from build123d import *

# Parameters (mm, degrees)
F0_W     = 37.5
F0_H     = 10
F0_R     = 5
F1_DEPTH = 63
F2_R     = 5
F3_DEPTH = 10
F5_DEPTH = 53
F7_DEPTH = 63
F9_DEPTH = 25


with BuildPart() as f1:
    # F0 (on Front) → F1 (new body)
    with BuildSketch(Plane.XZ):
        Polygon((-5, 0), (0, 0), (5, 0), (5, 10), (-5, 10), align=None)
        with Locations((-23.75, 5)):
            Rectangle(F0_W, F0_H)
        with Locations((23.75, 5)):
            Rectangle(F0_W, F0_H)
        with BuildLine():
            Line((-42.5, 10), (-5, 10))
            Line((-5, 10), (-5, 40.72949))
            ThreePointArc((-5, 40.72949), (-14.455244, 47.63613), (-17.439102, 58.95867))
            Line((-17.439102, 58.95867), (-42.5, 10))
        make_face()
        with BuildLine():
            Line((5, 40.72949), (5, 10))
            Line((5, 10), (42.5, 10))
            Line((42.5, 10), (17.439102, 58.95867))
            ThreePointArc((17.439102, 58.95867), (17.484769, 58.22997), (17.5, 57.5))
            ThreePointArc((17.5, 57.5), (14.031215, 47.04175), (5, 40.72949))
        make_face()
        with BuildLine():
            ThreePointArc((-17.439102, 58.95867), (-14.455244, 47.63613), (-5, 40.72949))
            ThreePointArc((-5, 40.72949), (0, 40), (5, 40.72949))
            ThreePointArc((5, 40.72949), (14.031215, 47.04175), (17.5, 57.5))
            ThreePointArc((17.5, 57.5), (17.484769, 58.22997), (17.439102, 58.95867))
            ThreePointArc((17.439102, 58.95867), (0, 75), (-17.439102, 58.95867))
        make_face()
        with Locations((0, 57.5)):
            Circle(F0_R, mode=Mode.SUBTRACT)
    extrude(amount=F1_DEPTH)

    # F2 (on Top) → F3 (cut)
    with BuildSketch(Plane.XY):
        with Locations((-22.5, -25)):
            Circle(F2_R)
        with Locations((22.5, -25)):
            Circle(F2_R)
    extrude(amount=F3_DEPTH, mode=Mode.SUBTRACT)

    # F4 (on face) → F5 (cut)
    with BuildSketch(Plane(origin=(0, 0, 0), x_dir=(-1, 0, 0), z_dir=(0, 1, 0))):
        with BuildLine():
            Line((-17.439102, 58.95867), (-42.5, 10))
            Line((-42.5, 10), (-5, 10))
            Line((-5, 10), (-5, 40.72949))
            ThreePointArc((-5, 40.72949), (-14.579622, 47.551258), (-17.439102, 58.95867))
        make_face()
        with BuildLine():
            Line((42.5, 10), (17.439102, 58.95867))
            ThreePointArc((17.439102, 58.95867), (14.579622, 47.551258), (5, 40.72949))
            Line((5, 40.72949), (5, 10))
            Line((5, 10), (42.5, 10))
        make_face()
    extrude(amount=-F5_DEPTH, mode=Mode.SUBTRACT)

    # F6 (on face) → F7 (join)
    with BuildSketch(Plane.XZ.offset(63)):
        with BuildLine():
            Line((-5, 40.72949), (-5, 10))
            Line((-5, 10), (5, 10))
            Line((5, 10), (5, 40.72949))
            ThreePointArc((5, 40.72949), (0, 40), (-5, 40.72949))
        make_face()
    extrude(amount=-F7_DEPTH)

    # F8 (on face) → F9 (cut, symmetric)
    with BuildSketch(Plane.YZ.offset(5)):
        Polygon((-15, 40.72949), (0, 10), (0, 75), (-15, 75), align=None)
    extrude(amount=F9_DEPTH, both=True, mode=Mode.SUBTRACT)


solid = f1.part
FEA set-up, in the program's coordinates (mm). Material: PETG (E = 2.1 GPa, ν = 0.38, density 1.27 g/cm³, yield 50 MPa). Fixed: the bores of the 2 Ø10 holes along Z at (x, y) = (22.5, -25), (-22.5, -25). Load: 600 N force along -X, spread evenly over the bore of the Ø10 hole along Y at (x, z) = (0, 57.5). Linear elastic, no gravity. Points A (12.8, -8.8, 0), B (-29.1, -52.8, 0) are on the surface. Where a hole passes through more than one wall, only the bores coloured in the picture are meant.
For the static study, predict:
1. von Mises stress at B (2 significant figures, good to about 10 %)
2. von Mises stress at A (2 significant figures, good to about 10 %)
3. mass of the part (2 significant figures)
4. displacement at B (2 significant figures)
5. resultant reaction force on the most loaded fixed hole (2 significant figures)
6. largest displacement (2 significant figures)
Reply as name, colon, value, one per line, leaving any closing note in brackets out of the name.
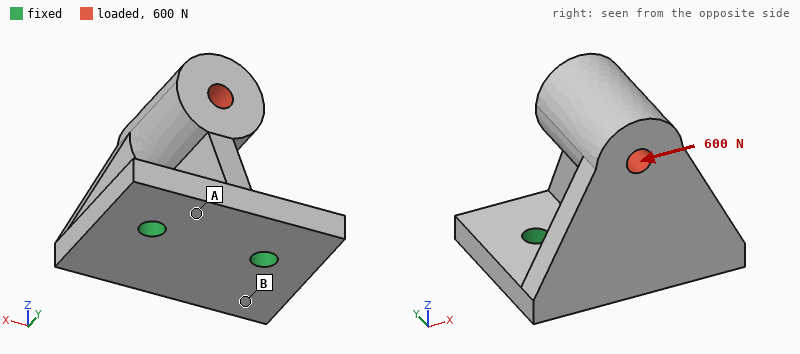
von Mises stress at B: 4.4 MPa
von Mises stress at A: 1.8 MPa
mass of the part: 170 g
displacement at B: 0.27 mm
resultant reaction force on the most loaded fixed hole: 760 N
largest displacement: 1.1 mm
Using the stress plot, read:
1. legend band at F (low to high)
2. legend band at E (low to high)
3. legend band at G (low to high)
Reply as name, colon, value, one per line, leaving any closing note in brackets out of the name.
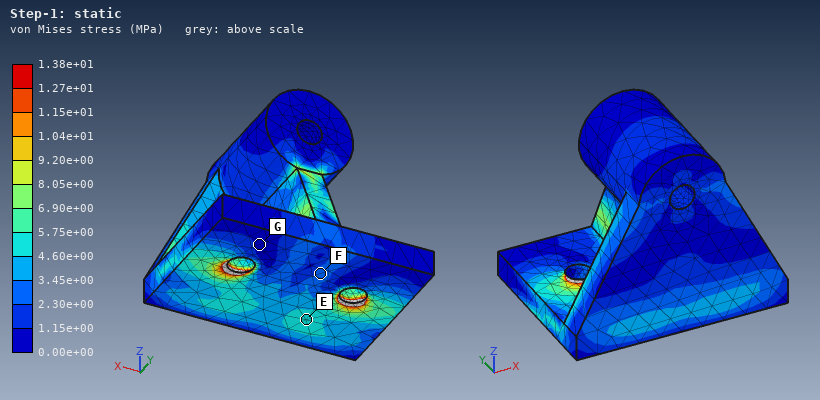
legend band at F: 2.30e+00 to 3.45e+00 MPa
legend band at E: 4.60e+00 to 5.75e+00 MPa
legend band at G: 0.00e+00 to 1.15e+00 MPa
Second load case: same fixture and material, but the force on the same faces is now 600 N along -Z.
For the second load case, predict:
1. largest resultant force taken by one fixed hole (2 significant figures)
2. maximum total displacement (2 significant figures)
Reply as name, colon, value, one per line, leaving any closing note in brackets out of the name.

largest resultant force taken by one fixed hole: 300 N
maximum total displacement: 0.29 mm
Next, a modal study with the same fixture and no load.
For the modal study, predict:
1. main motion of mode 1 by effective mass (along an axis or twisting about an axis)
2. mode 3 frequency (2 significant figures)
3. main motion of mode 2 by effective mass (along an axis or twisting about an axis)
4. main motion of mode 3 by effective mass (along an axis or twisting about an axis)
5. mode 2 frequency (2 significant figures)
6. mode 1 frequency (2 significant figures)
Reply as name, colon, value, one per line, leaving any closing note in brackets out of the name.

main motion of mode 1 by effective mass: along Y
mode 3 frequency: 1400 Hz
main motion of mode 2 by effective mass: along X
main motion of mode 3 by effective mass: twisting about Z
mode 2 frequency: 550 Hz
mode 1 frequency: 450 Hz
